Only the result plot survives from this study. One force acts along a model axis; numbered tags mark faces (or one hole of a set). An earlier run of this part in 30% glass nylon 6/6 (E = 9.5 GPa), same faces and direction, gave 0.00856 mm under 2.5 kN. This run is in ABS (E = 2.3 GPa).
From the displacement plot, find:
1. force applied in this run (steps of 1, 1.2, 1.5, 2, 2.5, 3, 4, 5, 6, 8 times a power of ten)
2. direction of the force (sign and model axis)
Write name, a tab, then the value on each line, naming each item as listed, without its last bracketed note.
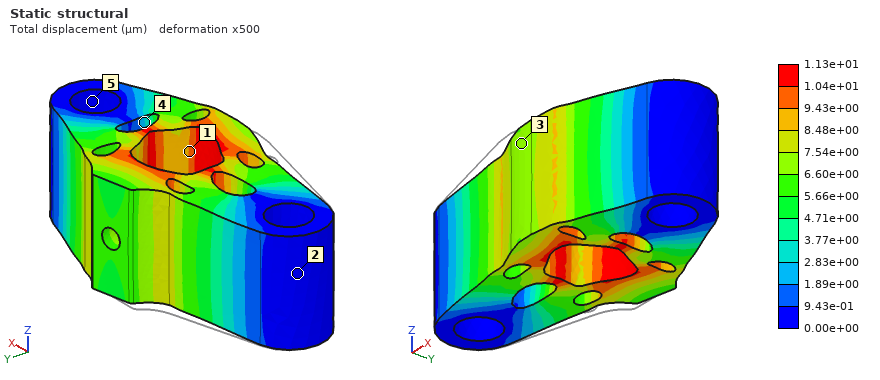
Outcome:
force applied in this run	800 N
direction of the force	+X
